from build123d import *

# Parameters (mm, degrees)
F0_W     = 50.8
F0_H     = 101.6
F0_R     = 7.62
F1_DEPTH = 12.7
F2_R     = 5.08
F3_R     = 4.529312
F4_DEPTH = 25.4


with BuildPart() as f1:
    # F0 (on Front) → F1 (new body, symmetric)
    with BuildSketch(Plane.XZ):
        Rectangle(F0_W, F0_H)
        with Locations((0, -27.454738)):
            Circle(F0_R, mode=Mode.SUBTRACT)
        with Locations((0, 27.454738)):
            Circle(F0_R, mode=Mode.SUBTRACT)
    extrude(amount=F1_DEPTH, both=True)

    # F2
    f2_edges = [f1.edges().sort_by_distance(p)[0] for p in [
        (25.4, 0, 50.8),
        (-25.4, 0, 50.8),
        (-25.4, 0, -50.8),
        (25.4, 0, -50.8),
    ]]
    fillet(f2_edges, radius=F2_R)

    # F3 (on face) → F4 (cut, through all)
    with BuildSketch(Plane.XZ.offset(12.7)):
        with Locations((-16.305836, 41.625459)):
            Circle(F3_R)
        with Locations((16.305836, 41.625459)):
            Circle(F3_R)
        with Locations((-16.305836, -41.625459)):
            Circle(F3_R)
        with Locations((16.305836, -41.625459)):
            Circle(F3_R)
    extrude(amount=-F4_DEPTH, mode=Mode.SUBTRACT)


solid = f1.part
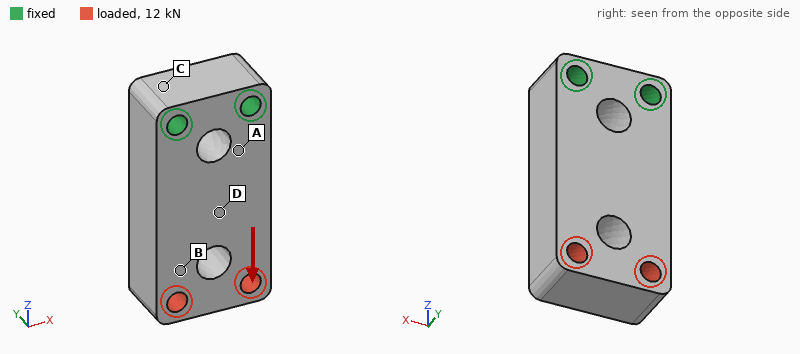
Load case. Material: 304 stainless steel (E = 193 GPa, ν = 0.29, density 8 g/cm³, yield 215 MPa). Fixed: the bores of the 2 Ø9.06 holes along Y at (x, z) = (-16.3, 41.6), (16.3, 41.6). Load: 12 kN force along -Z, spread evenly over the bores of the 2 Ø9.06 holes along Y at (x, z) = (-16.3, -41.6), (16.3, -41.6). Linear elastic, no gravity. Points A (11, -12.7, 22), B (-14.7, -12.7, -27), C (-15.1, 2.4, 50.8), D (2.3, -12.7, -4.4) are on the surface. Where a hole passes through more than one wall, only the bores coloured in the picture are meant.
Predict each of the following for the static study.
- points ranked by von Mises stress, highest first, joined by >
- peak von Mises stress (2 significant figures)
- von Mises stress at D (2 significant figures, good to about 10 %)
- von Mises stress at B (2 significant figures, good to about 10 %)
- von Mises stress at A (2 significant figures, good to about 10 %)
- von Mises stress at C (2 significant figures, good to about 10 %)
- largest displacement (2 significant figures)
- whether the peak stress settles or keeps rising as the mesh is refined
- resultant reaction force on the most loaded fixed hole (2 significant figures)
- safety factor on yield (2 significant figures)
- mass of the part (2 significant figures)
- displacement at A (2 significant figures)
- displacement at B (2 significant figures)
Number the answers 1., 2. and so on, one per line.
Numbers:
1. A > B > D > C
2. 31 MPa
3. 6.0 MPa
4. 9.7 MPa
5. 12 MPa
6. 2.7 MPa
7. 6.0 µm
8. settles
9. 6.0 kN
10. 6.9
11. 920 g
12. 1.2 µm
13. 3.9 µm
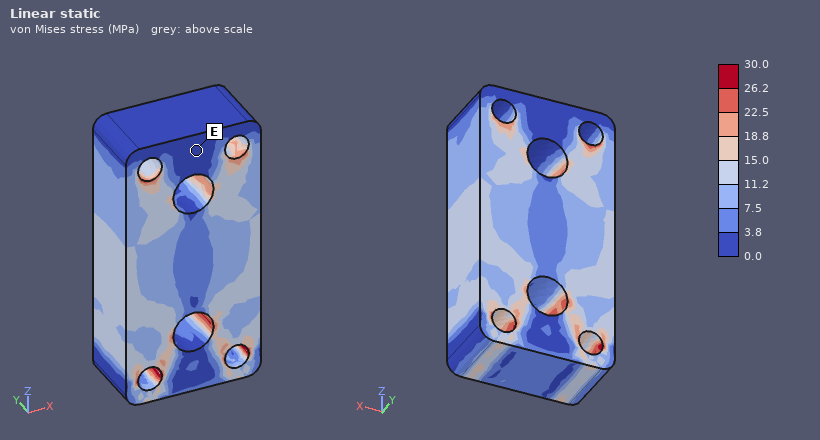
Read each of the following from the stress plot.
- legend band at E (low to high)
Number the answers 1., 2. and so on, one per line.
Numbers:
1. 0.0 to 3.8 MPa
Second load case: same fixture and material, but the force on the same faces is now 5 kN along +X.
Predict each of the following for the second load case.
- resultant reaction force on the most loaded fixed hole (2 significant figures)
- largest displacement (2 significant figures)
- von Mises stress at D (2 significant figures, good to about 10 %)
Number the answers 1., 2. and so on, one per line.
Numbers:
1. 11 kN
2. 29 µm
3. 14 MPa
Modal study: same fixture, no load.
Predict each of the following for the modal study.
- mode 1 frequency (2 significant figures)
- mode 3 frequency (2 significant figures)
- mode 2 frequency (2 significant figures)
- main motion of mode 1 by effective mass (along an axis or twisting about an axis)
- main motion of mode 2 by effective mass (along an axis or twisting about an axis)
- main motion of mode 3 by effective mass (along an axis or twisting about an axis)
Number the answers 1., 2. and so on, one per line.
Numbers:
1. 2300 Hz
2. 6500 Hz
3. 4100 Hz
4. along Y
5. along X
6. twisting about Z
